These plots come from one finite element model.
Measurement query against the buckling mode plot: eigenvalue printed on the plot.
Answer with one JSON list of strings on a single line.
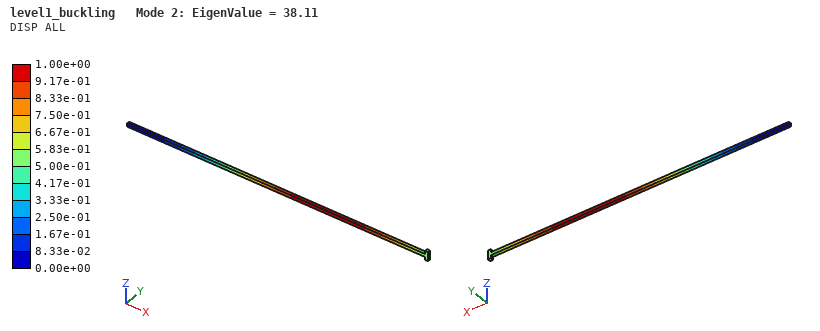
["38.11"]
